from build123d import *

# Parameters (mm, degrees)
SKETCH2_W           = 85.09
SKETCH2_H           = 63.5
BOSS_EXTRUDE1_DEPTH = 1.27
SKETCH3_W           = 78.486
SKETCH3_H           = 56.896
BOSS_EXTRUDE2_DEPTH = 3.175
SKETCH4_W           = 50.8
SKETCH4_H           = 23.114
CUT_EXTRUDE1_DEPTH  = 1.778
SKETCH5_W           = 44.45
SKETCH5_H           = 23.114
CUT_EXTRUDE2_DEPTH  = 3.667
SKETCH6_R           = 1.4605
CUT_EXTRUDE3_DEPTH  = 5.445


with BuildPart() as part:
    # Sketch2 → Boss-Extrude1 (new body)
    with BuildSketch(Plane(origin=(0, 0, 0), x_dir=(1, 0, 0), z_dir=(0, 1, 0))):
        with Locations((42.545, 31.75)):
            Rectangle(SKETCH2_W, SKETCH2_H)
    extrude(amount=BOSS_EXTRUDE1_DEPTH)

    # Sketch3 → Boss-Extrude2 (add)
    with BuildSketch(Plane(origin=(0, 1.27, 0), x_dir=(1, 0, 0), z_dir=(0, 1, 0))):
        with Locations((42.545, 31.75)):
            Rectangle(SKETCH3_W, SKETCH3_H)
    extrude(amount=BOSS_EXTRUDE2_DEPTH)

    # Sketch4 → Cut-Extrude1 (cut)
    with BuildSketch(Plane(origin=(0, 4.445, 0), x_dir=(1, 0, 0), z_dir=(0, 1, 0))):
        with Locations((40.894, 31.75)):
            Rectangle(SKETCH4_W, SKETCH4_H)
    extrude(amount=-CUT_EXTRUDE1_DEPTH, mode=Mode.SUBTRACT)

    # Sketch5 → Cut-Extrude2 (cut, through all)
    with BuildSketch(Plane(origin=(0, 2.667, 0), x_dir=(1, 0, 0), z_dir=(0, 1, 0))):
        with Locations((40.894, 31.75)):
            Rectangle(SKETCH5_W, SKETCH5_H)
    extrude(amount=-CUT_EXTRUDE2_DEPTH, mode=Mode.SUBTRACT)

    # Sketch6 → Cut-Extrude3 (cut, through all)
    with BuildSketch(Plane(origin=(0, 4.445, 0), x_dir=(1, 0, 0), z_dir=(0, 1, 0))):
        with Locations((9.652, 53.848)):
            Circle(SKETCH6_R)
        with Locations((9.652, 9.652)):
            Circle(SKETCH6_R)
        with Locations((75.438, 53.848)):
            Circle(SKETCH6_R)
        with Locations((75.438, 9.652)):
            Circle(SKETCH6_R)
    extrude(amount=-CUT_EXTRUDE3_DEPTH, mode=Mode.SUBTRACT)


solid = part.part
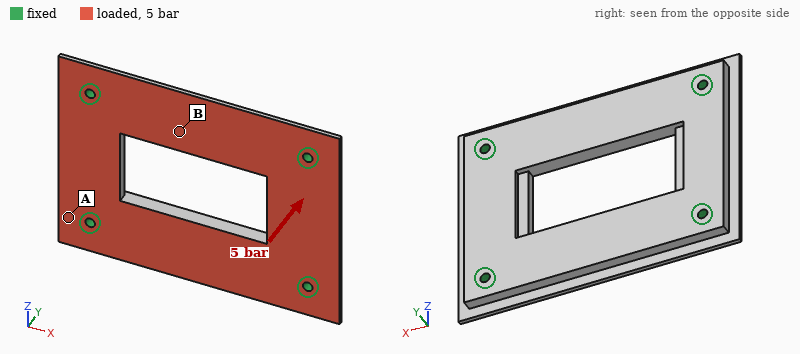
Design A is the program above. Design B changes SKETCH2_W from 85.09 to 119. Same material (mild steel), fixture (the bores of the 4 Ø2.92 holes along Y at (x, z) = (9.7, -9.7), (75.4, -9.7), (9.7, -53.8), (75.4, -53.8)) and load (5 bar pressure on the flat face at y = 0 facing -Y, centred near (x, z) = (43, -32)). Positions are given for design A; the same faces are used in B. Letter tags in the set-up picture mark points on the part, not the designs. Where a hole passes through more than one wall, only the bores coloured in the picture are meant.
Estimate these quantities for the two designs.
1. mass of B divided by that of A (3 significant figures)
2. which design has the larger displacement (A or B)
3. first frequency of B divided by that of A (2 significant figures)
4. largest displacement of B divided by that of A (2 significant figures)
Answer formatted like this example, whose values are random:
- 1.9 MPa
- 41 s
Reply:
- 1.17
- B
- 0.49
- 15
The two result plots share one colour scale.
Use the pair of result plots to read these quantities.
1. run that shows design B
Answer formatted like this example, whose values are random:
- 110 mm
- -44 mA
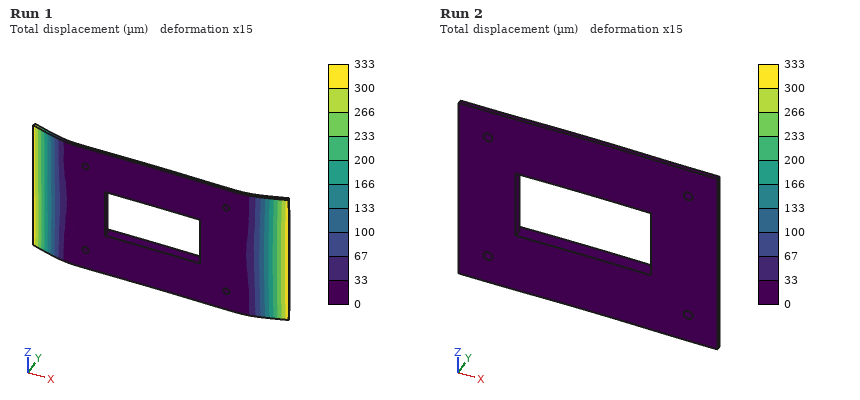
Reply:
- Run 1
